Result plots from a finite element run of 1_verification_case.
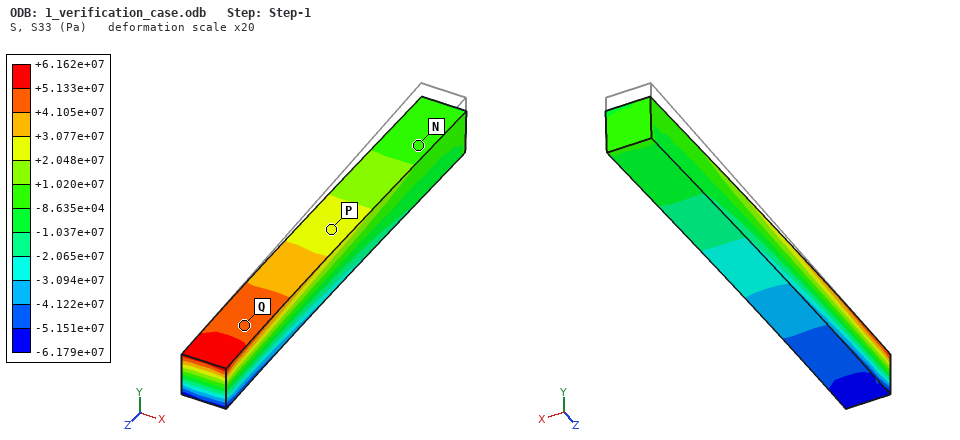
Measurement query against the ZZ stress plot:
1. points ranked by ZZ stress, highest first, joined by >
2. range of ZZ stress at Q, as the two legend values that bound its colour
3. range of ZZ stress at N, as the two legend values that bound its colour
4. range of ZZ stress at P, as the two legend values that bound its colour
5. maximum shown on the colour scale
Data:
Q > P > N
+4.105e+07 to +5.133e+07 Pa
-8.635e+04 to +1.020e+07 Pa
+2.048e+07 to +3.077e+07 Pa
+6.162e+07 Pa
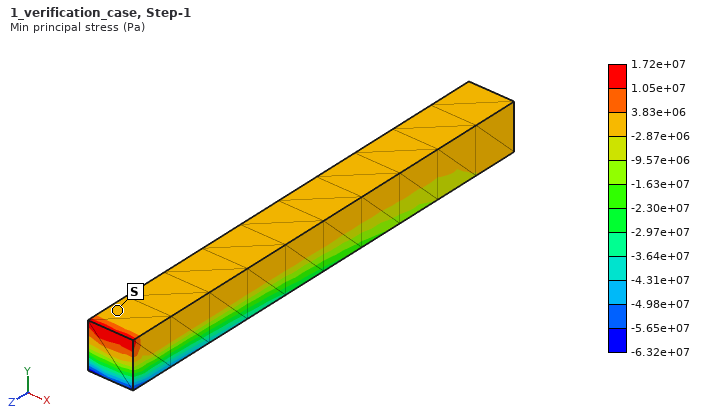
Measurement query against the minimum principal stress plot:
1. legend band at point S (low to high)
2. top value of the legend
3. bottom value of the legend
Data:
-2.87e+06 to 3.83e+06 Pa
1.72e+07 Pa
-6.32e+07 Pa
